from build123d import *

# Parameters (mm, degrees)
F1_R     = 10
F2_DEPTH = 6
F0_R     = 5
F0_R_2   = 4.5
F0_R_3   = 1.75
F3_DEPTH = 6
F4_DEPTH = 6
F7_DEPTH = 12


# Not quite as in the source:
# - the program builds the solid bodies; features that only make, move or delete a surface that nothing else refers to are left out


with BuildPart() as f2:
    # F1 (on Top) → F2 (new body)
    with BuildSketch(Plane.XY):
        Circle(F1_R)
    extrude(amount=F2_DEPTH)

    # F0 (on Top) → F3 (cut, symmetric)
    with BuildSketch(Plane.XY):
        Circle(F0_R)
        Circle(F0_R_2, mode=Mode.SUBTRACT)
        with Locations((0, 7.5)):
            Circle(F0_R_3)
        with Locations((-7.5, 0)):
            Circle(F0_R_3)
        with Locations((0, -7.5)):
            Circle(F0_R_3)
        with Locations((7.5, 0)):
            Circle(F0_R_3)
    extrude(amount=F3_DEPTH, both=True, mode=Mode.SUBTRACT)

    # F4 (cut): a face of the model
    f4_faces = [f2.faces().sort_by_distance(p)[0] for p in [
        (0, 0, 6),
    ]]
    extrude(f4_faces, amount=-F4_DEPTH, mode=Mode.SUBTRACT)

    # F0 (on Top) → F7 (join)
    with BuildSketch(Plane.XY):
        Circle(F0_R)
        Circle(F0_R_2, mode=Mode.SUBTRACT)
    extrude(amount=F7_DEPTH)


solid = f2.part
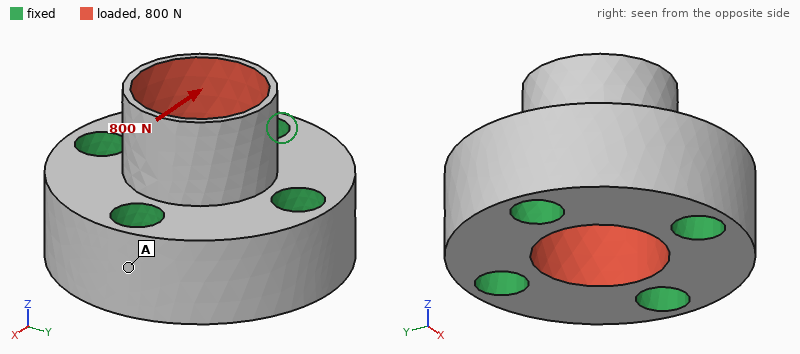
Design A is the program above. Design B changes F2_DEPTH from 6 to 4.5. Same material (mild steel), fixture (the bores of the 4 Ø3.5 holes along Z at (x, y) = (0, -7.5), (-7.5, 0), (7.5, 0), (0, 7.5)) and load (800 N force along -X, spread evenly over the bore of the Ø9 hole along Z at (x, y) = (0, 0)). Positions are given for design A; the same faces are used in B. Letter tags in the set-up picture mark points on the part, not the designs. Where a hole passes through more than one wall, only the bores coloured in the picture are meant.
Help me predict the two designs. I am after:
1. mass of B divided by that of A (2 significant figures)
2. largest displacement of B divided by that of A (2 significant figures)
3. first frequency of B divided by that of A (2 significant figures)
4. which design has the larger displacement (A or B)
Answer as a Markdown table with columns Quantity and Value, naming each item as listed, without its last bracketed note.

| Quantity | Value |
|---|---|
| mass of B divided by that of A | 0.78 |
| largest displacement of B divided by that of A | 1.6 |
| first frequency of B divided by that of A | 0.75 |
| which design has the larger displacement | B |
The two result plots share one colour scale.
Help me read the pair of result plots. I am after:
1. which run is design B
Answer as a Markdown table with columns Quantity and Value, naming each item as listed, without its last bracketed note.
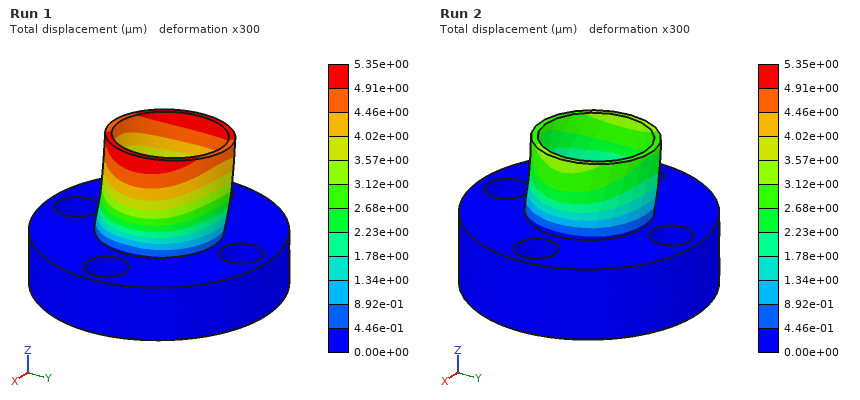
| Quantity | Value |
|---|---|
| which run is design B | Run 1 |
